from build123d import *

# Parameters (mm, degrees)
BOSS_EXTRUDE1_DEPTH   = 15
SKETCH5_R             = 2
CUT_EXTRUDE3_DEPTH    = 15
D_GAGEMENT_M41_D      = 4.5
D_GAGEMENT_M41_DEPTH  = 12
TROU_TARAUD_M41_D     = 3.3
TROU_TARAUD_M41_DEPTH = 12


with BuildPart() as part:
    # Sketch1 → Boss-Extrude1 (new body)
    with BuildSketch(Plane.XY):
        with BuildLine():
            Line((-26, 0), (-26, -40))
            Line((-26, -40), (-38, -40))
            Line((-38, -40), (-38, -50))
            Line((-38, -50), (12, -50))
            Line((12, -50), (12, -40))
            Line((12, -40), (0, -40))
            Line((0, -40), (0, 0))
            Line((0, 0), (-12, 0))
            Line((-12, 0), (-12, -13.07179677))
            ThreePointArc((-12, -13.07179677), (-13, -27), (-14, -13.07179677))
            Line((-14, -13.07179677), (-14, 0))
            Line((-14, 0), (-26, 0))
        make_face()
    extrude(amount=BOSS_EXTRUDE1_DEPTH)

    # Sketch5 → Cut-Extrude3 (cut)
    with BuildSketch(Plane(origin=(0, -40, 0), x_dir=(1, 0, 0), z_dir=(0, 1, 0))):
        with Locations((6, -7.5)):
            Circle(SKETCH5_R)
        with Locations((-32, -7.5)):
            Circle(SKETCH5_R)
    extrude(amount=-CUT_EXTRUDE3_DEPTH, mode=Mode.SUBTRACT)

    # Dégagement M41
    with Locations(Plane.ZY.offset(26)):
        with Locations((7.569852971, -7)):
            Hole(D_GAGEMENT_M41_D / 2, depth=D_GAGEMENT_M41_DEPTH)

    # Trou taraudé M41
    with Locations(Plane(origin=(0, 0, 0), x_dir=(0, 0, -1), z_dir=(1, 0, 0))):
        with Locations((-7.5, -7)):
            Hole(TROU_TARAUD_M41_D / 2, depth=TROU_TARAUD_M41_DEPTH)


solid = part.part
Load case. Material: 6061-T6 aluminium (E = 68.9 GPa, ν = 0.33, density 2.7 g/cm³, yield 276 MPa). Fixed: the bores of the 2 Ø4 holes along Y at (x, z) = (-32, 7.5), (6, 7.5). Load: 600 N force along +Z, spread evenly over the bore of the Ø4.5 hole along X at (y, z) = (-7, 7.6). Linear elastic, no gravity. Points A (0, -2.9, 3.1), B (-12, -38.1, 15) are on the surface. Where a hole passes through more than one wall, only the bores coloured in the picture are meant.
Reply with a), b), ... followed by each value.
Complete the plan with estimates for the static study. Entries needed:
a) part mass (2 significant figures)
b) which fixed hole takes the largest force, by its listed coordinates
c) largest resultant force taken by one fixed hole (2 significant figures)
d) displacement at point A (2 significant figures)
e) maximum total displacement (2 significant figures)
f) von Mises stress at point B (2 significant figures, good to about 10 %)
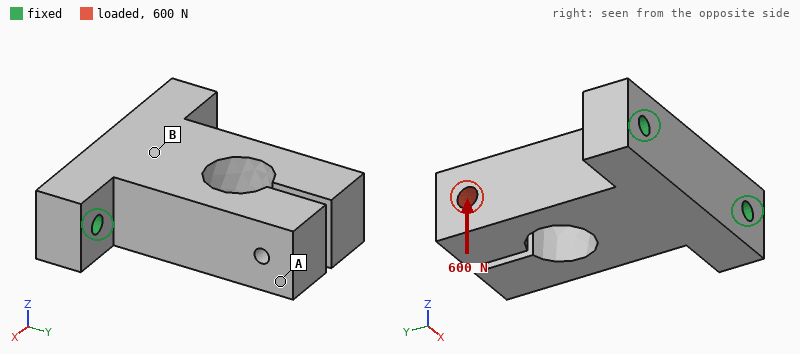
a) 54 g
b) (-32, 7.5)
c) 410 N
d) 0.062 mm
e) 0.13 mm
f) 16 MPa
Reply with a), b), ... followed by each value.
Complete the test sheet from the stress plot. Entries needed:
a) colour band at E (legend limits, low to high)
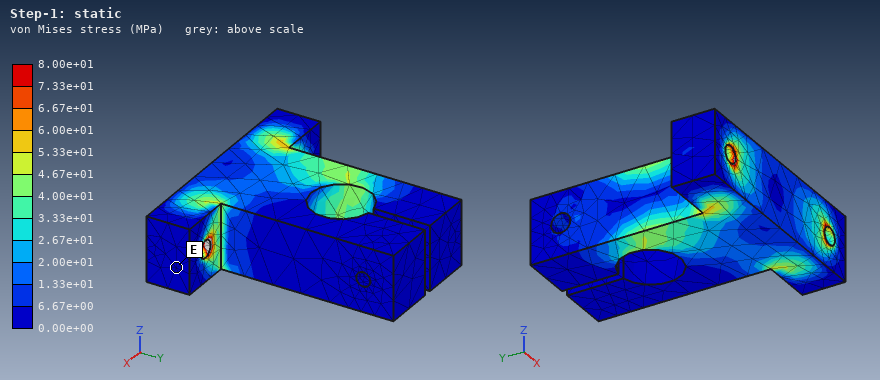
a) 0.00e+00 to 6.67e+00 MPa
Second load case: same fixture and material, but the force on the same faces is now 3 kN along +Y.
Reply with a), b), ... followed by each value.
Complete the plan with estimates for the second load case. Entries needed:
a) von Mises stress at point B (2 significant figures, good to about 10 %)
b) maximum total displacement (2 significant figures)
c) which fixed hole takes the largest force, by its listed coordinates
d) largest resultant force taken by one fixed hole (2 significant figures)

a) 7.6 MPa
b) 0.10 mm
c) (-32, 7.5)
d) 2.2 kN
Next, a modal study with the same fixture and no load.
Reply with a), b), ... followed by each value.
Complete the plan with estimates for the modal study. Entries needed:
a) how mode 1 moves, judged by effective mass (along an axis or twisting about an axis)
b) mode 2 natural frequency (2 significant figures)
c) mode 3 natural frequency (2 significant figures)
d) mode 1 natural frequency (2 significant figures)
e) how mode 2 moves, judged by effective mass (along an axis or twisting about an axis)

a) along Z
b) 4500 Hz
c) 4900 Hz
d) 3400 Hz
e) along X
